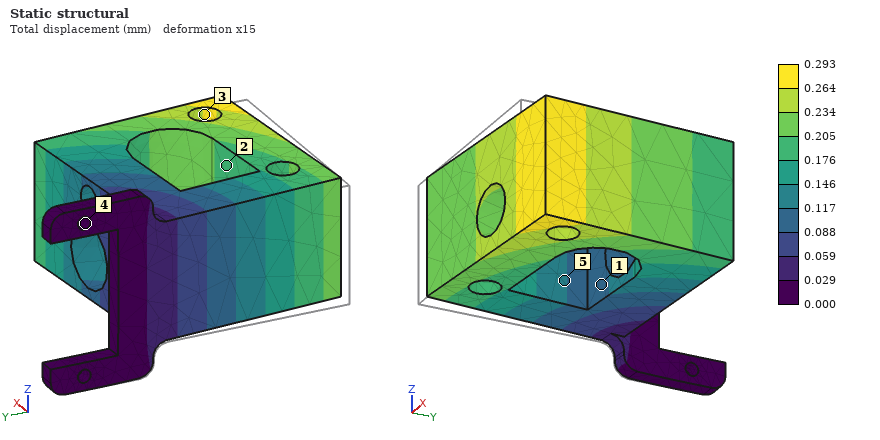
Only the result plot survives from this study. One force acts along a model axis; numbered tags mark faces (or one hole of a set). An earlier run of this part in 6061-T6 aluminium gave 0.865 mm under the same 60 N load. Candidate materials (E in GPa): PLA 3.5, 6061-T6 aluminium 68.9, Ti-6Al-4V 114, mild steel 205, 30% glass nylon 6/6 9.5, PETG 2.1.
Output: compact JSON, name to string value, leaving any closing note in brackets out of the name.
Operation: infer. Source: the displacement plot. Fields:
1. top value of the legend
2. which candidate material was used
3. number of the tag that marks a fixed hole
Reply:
{"top value of the legend": "0.293 mm", "which candidate material was used": "mild steel", "number of the tag that marks a fixed hole": "4"}
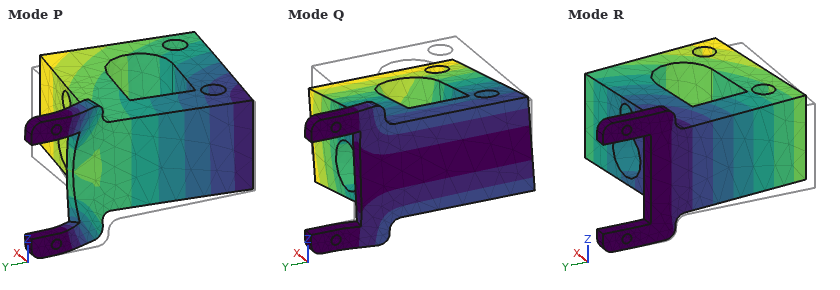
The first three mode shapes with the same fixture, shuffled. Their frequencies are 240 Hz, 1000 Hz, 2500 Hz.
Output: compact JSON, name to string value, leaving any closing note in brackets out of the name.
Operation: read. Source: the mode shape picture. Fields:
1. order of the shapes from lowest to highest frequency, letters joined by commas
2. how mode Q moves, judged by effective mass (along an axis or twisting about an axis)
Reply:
{"order of the shapes from lowest to highest frequency, letters joined by commas": "R, Q, P", "how mode Q moves, judged by effective mass": "along Z"}
